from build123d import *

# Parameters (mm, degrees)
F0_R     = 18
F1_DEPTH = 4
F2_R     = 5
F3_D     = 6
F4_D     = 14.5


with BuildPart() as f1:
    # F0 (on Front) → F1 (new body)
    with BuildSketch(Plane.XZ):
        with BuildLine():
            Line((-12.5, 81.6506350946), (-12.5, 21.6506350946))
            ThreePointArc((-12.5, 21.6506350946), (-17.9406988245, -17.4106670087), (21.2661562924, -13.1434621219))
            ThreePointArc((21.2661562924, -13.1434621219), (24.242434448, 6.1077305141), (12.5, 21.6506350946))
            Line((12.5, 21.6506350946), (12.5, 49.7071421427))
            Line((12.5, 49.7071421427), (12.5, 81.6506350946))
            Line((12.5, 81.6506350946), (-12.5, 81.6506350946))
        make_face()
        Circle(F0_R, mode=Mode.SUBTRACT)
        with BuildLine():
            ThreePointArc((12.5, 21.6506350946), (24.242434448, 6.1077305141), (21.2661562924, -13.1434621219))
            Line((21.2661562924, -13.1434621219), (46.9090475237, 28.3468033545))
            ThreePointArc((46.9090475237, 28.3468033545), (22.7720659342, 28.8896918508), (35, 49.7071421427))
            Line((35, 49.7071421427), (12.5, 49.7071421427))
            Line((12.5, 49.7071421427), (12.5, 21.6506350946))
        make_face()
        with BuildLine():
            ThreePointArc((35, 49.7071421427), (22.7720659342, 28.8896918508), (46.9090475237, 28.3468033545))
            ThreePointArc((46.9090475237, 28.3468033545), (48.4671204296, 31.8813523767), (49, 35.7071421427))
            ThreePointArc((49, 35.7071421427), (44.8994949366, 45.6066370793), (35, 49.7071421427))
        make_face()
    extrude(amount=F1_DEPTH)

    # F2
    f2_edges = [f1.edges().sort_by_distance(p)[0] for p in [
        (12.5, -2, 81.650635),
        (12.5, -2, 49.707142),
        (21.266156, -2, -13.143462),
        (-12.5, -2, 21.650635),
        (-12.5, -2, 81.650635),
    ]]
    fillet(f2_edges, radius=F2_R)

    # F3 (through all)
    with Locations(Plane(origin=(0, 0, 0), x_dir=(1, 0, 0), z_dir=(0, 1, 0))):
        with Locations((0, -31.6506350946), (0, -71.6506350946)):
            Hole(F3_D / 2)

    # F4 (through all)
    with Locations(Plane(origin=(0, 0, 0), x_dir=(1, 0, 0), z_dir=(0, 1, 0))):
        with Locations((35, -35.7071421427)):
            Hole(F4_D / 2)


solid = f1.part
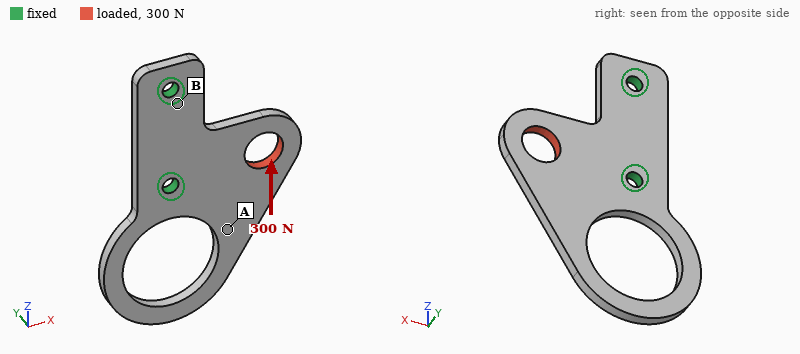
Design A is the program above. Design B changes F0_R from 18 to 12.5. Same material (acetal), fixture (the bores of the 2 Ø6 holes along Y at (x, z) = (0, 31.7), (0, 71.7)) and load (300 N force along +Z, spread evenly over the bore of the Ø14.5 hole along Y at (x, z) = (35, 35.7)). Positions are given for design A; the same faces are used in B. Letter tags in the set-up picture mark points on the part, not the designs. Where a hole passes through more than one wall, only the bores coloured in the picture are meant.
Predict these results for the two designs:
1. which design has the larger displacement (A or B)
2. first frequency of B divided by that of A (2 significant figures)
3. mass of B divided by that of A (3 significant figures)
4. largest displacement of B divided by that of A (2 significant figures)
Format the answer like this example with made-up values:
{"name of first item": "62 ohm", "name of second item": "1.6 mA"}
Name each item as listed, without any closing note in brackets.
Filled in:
{"which design has the larger displacement": "A", "first frequency of B divided by that of A": "1.0", "mass of B divided by that of A": "1.15", "largest displacement of B divided by that of A": "0.91"}
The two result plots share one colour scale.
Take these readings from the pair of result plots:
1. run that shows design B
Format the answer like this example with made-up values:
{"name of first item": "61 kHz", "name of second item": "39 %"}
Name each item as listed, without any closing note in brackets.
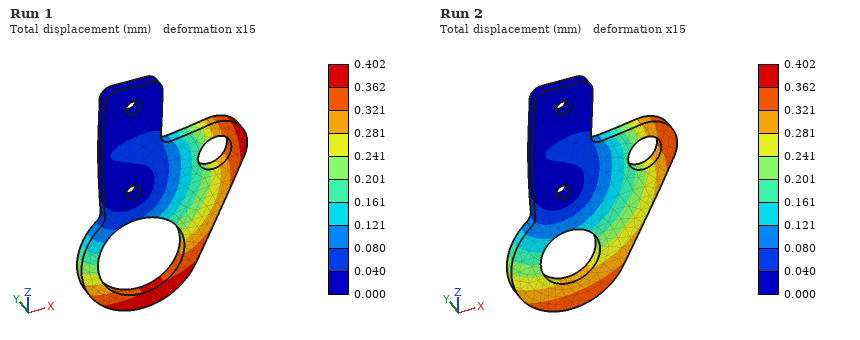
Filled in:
{"run that shows design B": "Run 2"}
